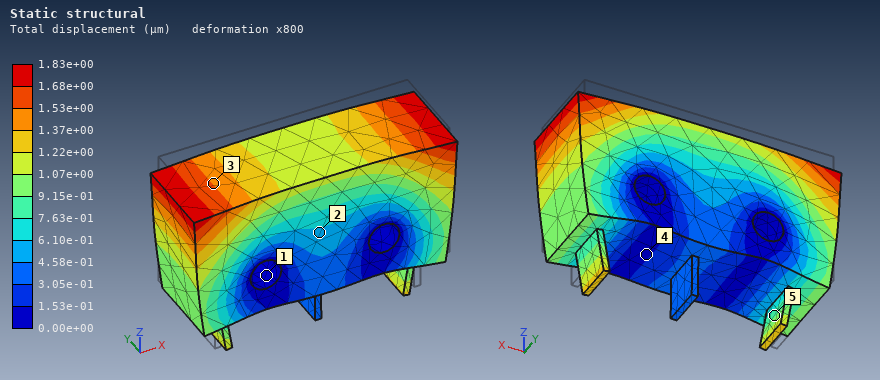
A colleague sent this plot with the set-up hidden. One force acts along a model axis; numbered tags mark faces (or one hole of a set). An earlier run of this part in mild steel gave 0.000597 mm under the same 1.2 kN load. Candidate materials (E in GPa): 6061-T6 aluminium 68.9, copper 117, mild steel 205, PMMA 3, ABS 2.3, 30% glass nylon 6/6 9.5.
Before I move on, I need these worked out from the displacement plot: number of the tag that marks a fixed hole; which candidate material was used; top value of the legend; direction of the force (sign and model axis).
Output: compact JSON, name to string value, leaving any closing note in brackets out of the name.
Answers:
{"number of the tag that marks a fixed hole": "1", "which candidate material was used": "6061-T6 aluminium", "top value of the legend": "1.83e+00 µm", "direction of the force": "-Z"}
